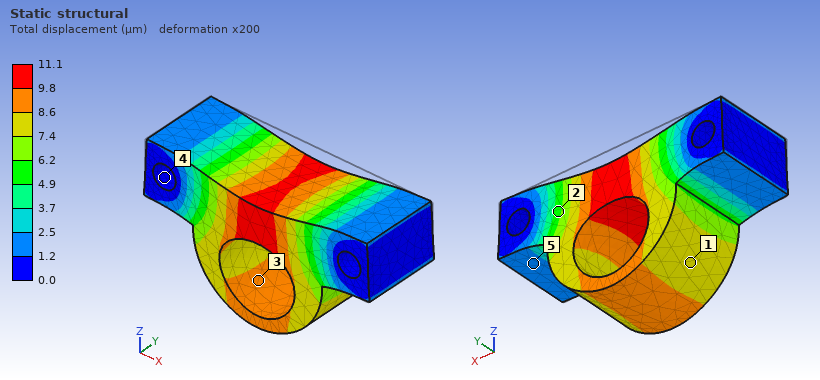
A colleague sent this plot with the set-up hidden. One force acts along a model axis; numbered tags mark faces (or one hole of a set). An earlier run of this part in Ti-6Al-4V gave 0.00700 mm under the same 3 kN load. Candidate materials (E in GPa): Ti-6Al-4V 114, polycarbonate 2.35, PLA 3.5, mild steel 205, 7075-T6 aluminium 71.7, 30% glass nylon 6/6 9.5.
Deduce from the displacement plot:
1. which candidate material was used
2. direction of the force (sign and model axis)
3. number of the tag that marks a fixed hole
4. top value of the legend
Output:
7075-T6 aluminium
-Z
4
11.1 µm
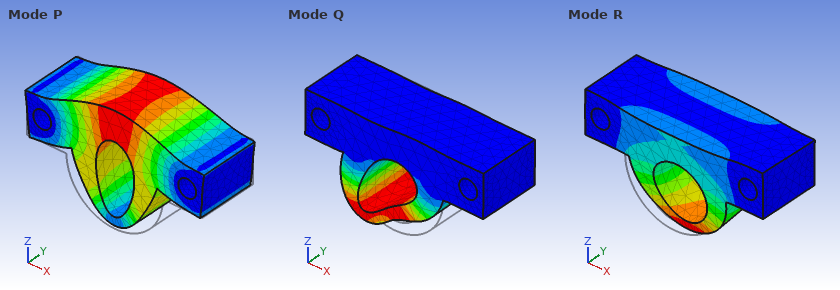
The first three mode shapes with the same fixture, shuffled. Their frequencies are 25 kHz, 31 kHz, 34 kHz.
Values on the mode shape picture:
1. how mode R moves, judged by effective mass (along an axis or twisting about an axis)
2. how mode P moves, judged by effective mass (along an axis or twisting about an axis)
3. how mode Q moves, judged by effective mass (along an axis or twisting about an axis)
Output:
along Y
along Z
along X
